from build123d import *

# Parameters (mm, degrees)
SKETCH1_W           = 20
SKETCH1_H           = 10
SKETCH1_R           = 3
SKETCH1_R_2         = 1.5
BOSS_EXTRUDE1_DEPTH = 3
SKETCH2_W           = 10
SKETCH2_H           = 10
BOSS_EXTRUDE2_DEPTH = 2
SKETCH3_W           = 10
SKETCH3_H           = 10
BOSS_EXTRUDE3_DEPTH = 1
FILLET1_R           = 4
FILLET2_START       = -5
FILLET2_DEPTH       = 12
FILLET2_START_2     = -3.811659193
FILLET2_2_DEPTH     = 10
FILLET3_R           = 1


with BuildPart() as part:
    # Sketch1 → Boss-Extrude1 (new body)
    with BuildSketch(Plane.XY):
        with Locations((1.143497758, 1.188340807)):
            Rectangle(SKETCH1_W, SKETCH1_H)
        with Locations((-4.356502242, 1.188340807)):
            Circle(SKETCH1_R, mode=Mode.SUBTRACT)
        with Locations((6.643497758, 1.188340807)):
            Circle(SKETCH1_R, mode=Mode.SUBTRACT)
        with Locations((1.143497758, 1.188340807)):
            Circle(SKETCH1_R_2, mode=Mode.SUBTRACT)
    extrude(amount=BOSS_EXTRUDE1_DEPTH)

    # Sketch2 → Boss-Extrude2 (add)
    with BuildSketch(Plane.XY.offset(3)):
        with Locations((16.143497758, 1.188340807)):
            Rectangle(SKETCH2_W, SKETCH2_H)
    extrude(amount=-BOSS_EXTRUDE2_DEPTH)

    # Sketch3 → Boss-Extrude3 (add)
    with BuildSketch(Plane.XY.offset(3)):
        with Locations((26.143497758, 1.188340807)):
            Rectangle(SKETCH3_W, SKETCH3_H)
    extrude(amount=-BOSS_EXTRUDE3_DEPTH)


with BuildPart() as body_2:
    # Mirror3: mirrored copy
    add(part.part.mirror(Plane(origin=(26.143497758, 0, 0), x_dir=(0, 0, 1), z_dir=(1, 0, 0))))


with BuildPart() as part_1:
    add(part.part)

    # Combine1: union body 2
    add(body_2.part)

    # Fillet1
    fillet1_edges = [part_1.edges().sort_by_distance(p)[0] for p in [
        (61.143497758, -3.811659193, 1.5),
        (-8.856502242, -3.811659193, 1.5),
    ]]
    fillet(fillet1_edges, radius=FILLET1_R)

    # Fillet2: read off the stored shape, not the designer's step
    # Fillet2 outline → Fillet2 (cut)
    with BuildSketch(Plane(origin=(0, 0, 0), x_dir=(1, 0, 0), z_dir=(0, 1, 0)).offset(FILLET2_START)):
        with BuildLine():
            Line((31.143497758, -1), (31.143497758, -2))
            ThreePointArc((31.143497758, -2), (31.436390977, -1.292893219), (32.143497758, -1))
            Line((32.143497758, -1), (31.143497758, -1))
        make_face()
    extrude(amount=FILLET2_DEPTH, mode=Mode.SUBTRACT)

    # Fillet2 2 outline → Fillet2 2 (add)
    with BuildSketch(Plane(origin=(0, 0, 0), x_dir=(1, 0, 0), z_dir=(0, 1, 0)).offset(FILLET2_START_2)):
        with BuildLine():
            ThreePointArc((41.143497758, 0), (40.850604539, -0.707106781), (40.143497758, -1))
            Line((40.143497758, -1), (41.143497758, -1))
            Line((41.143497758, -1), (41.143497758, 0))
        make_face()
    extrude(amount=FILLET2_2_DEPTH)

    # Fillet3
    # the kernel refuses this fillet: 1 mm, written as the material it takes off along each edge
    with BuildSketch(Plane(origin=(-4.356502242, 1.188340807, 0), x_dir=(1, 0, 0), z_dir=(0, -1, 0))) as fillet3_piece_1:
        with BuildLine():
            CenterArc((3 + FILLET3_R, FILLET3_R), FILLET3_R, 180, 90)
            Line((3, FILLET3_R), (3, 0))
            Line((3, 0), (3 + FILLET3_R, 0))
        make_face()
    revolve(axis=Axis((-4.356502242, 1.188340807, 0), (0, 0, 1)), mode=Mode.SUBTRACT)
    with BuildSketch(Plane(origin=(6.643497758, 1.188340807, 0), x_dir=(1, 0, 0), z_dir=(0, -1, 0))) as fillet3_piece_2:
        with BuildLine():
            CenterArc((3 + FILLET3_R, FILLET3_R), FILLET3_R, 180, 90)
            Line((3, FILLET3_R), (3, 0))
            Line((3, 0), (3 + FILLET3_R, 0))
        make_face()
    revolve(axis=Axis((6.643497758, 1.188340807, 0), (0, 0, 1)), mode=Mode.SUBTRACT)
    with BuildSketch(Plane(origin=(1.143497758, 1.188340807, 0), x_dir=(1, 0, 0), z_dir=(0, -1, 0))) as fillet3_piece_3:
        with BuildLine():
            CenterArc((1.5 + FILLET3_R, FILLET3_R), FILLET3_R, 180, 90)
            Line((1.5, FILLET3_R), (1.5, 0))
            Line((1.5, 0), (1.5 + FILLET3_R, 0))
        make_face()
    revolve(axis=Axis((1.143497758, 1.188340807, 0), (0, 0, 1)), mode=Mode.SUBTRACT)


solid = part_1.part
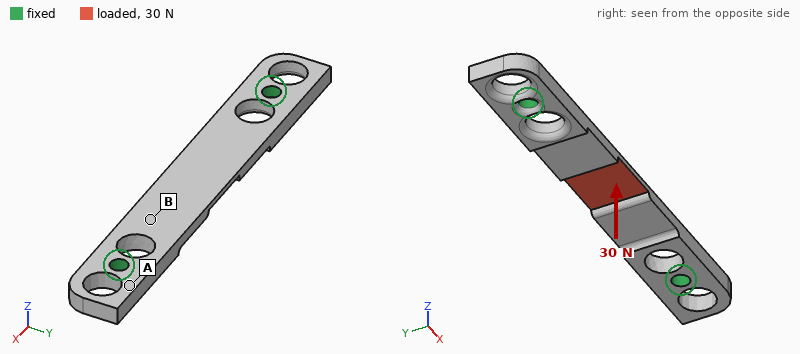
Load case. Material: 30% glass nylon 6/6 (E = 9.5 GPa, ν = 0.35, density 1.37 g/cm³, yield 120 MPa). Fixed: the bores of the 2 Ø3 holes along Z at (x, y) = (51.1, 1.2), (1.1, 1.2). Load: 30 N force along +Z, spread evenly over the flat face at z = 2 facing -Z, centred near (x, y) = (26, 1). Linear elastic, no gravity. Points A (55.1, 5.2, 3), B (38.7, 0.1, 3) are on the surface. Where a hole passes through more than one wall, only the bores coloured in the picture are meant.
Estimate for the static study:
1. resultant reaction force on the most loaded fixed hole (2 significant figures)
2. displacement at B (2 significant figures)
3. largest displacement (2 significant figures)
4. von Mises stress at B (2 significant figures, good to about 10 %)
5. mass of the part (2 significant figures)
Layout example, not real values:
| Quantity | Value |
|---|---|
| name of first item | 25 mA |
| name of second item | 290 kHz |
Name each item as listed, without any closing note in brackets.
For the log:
| Quantity | Value |
|---|---|
| resultant reaction force on the most loaded fixed hole | 74 N |
| displacement at B | 0.12 mm |
| largest displacement | 0.34 mm |
| von Mises stress at B | 8.2 MPa |
| mass of the part | 1.8 g |
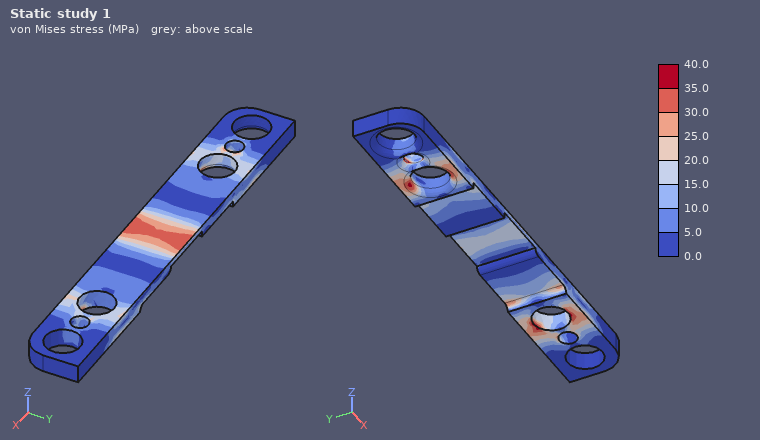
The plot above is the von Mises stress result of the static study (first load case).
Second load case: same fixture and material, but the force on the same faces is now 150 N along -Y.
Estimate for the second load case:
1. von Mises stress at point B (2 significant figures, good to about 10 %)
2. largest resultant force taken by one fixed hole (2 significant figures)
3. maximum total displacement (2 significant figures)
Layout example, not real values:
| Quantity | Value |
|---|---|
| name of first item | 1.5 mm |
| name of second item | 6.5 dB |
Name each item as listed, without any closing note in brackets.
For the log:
| Quantity | Value |
|---|---|
| von Mises stress at point B | 12 MPa |
| largest resultant force taken by one fixed hole | 77 N |
| maximum total displacement | 0.18 mm |
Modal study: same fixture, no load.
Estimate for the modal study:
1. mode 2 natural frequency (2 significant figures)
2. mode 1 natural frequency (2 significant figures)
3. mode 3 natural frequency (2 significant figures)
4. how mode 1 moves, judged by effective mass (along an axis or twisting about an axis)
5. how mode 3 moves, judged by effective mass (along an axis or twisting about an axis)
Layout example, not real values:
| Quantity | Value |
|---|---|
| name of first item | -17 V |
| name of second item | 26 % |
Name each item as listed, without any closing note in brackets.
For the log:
| Quantity | Value |
|---|---|
| mode 2 natural frequency | 5400 Hz |
| mode 1 natural frequency | 2600 Hz |
| mode 3 natural frequency | 6300 Hz |
| how mode 1 moves, judged by effective mass | along Z |
| how mode 3 moves, judged by effective mass | along Y |
